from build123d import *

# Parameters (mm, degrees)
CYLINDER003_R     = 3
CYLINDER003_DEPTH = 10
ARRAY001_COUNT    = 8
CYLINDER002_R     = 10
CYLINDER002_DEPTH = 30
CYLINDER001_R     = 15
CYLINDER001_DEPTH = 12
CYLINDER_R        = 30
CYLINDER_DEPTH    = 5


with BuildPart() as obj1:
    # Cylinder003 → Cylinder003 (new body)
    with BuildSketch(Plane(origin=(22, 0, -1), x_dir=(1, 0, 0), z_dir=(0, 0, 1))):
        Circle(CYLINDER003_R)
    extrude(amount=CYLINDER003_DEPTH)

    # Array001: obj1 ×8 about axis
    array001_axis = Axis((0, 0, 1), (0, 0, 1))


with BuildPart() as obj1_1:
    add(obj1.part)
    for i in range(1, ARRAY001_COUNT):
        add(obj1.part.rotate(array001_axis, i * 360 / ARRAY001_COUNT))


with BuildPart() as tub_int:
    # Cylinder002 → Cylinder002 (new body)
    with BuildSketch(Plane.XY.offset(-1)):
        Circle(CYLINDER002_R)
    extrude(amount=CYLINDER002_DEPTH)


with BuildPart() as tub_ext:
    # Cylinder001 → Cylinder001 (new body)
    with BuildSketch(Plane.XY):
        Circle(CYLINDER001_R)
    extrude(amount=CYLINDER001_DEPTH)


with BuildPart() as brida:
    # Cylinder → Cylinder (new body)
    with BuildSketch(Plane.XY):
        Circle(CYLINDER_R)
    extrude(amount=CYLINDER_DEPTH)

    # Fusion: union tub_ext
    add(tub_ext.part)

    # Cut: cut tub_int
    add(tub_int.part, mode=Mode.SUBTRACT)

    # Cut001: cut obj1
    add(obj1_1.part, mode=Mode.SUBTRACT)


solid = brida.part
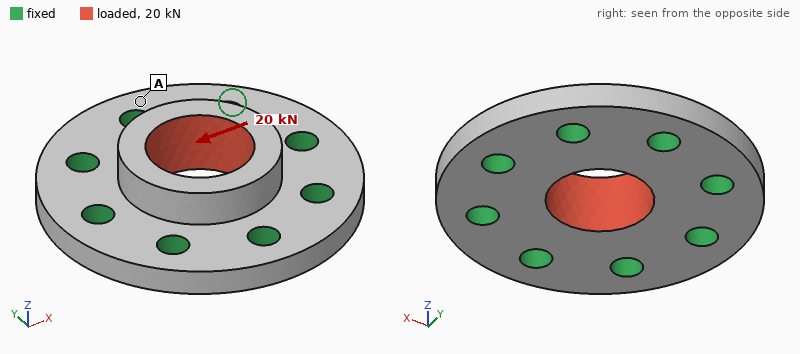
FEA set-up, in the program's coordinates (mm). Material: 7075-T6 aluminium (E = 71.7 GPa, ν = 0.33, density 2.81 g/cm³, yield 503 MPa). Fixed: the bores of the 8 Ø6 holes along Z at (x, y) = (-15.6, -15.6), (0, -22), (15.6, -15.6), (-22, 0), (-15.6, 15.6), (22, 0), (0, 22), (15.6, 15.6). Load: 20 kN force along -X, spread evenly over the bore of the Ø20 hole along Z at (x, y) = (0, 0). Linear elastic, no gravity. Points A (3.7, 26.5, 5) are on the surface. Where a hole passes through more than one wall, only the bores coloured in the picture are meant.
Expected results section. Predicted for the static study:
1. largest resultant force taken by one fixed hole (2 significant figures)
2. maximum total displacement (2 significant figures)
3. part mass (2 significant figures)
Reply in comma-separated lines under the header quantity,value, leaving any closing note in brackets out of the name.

quantity,value
largest resultant force taken by one fixed hole,3.9 kN
maximum total displacement,26 µm
part mass,40 g
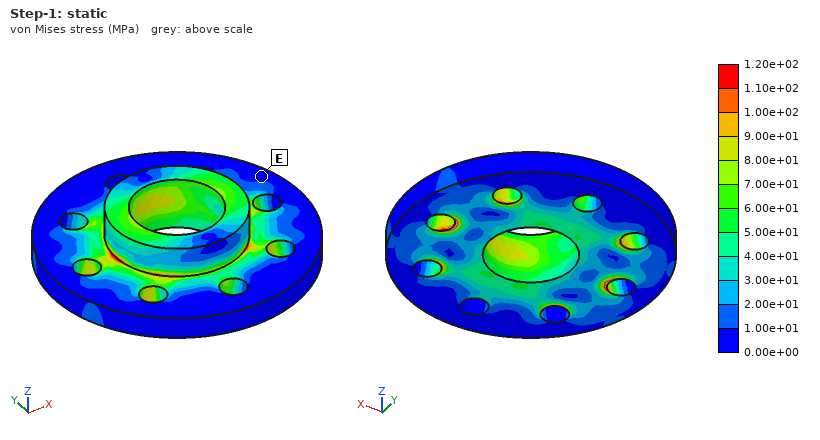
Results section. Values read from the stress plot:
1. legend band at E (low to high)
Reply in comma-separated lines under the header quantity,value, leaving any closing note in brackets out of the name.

quantity,value
legend band at E,0.00e+00 to 1.00e+01 MPa
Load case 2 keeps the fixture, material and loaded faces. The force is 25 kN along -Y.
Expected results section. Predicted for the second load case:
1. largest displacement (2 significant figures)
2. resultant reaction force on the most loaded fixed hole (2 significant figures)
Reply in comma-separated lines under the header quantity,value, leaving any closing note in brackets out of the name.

quantity,value
largest displacement,32 µm
resultant reaction force on the most loaded fixed hole,4.8 kN
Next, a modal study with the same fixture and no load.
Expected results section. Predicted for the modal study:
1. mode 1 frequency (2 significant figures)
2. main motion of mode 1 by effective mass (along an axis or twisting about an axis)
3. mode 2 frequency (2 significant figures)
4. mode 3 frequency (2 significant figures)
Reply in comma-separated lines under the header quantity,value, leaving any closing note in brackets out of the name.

quantity,value
mode 1 frequency,36 kHz
main motion of mode 1 by effective mass,along Z
mode 2 frequency,44 kHz
mode 3 frequency,44 kHz
